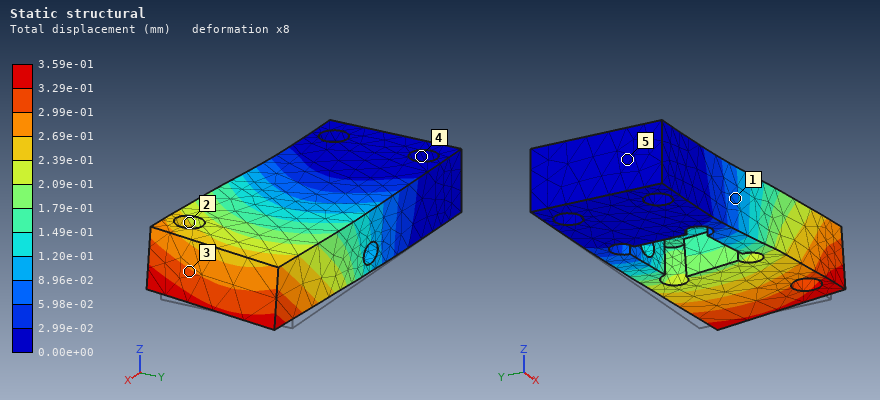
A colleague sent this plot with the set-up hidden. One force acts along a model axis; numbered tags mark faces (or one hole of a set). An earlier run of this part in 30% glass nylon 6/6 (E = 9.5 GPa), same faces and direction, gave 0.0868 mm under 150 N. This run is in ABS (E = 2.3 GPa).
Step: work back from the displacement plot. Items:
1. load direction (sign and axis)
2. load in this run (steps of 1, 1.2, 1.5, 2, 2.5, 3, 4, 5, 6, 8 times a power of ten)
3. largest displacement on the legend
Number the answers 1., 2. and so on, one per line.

1. -Y
2. 150 N
3. 3.59e-01 mm
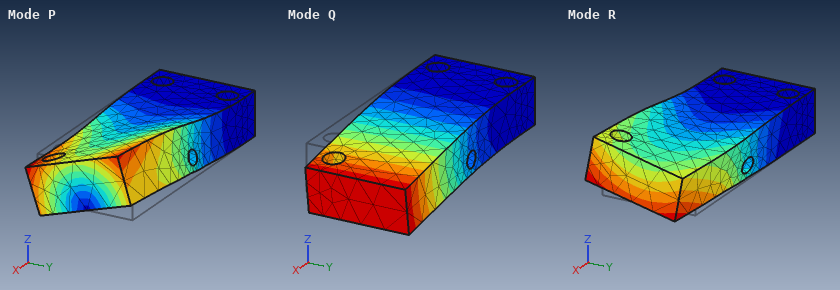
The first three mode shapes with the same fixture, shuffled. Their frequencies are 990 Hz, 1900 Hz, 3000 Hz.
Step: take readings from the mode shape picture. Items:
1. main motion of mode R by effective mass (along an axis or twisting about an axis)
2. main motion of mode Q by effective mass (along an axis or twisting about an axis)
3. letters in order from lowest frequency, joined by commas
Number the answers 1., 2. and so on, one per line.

1. along Y
2. along Z
3. Q, R, P
